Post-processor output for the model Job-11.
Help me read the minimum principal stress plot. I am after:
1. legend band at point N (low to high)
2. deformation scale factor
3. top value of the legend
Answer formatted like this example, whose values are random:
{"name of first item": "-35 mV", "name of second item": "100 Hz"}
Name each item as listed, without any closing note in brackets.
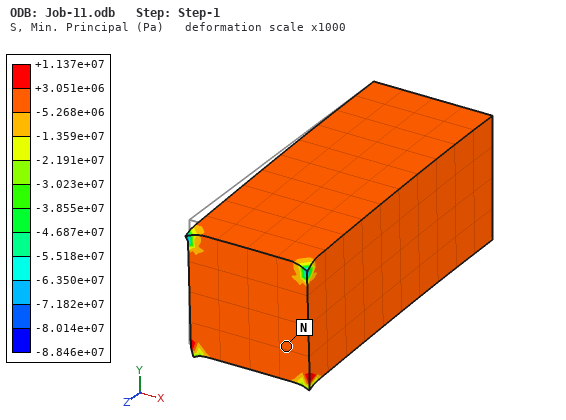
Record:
{"legend band at point N": "-5.268e+06 to +3.051e+06 Pa", "deformation scale factor": "1000", "top value of the legend": "+1.137e+07 Pa"}
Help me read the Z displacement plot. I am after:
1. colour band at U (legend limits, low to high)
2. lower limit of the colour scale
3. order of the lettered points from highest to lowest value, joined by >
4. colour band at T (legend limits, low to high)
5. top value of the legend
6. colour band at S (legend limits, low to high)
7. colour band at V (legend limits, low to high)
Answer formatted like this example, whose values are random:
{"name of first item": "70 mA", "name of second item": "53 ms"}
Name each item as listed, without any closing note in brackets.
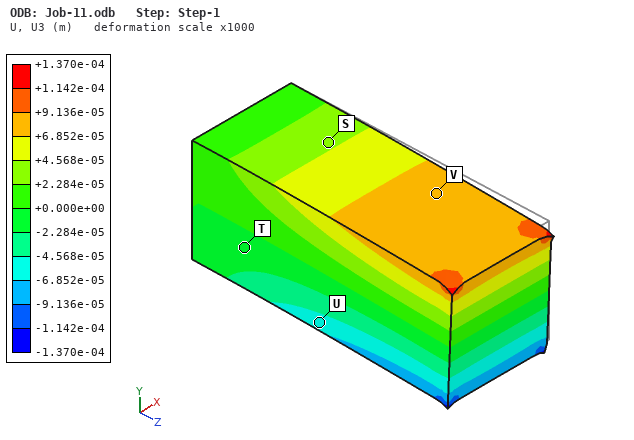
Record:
{"colour band at U": "-6.852e-05 to -4.568e-05 m", "lower limit of the colour scale": "-1.370e-04 m", "order of the lettered points from highest to lowest value, joined by >": "V > S > T > U", "colour band at T": "-2.284e-05 to +0.000e+00 m", "top value of the legend": "+1.370e-04 m", "colour band at S": "+2.284e-05 to +4.568e-05 m", "colour band at V": "+6.852e-05 to +9.136e-05 m"}
